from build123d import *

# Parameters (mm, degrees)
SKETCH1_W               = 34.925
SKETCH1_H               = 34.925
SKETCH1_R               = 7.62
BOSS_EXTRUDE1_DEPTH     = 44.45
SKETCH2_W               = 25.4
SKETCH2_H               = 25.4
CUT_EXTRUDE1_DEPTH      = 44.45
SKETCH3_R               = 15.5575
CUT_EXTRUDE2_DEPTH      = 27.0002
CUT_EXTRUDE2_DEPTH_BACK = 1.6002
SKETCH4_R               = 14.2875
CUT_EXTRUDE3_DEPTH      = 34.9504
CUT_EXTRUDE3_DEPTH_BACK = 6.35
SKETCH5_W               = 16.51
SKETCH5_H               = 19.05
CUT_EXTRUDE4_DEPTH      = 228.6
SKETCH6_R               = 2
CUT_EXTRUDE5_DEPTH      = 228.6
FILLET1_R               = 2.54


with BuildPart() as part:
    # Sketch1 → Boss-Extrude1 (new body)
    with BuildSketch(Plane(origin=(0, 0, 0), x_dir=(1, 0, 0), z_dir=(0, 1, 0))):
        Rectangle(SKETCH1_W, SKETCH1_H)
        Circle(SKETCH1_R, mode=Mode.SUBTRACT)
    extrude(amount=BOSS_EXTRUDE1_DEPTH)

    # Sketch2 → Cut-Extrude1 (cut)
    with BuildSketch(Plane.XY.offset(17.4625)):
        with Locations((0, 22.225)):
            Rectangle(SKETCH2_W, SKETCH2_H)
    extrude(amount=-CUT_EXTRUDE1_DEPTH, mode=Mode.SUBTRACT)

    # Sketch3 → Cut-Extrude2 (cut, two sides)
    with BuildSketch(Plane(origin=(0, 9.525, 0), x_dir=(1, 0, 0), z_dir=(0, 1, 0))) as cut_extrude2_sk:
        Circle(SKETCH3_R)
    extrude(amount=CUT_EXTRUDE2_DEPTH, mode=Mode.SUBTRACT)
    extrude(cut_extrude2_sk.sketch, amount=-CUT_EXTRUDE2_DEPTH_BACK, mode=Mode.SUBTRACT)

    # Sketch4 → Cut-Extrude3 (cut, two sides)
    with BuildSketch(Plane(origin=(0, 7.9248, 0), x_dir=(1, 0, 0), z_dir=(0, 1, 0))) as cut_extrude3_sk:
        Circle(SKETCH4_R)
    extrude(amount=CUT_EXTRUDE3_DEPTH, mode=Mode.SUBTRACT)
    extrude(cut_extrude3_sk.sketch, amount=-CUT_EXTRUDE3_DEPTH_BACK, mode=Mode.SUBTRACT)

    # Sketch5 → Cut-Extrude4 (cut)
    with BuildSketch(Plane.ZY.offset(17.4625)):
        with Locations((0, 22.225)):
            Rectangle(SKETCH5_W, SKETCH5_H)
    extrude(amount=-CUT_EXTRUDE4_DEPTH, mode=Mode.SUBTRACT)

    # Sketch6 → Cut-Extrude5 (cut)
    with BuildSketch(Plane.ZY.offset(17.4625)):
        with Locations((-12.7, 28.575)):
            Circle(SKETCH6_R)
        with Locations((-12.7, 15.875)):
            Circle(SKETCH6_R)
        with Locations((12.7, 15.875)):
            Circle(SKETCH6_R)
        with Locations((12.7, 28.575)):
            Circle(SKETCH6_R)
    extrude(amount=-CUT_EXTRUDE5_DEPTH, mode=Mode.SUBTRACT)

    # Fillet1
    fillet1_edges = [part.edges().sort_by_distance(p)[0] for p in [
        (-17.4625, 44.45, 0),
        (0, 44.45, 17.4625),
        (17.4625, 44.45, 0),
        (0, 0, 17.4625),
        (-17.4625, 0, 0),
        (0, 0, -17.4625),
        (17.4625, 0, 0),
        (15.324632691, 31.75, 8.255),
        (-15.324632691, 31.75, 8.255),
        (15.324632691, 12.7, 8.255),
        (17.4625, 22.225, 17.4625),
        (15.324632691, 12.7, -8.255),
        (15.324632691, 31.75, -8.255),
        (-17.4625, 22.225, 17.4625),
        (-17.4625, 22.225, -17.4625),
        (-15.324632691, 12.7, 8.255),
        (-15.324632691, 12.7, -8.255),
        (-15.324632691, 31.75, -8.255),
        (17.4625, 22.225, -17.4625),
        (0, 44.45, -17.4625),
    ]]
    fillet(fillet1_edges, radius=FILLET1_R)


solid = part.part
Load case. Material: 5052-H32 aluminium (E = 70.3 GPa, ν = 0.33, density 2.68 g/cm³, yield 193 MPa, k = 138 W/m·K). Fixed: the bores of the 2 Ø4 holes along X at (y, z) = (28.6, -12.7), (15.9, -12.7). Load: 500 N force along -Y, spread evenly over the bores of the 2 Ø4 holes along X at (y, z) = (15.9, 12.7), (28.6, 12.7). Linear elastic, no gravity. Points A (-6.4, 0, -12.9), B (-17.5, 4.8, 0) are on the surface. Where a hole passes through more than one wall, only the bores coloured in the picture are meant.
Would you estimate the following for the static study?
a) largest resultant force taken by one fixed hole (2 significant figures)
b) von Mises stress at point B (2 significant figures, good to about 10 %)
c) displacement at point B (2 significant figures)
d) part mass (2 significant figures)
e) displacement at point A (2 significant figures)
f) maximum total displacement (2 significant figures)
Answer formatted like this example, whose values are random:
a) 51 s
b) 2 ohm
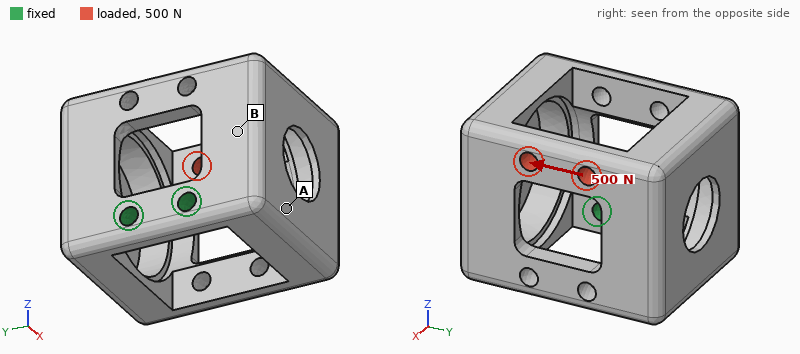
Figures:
a) 670 N
b) 20 MPa
c) 0.044 mm
d) 43 g
e) 0.074 mm
f) 0.19 mm
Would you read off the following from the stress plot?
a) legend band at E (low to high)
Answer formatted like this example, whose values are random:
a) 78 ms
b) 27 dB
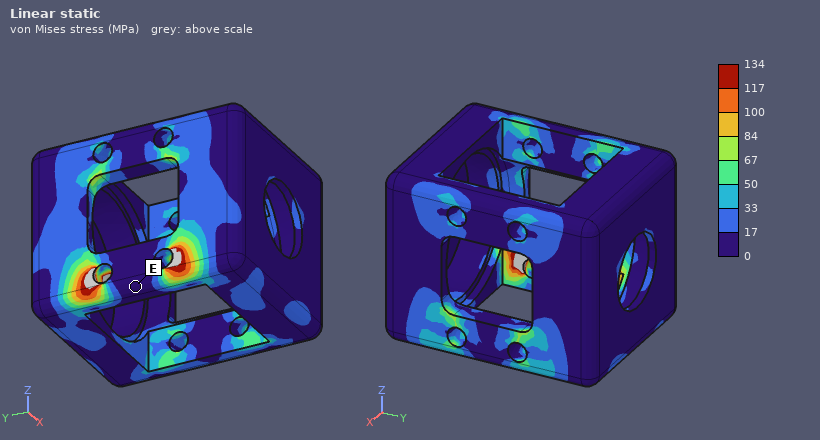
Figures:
a) 0 to 17 MPa
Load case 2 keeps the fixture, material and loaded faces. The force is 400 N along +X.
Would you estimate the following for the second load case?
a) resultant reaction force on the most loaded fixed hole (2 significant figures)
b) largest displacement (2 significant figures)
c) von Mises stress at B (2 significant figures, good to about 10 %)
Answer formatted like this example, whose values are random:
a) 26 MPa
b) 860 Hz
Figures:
a) 210 N
b) 0.26 mm
c) 23 MPa
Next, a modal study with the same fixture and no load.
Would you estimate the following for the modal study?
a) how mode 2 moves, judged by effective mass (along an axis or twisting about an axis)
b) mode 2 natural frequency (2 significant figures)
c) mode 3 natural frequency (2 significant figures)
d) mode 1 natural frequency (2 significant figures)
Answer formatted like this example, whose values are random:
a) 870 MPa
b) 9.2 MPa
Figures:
a) along Y
b) 1900 Hz
c) 3200 Hz
d) 1200 Hz
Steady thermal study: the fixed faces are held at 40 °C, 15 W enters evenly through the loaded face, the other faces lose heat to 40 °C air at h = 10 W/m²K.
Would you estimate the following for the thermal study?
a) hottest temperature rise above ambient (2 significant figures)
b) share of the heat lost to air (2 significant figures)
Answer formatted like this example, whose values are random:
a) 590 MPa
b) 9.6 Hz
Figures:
a) 42 K
b) 13 %
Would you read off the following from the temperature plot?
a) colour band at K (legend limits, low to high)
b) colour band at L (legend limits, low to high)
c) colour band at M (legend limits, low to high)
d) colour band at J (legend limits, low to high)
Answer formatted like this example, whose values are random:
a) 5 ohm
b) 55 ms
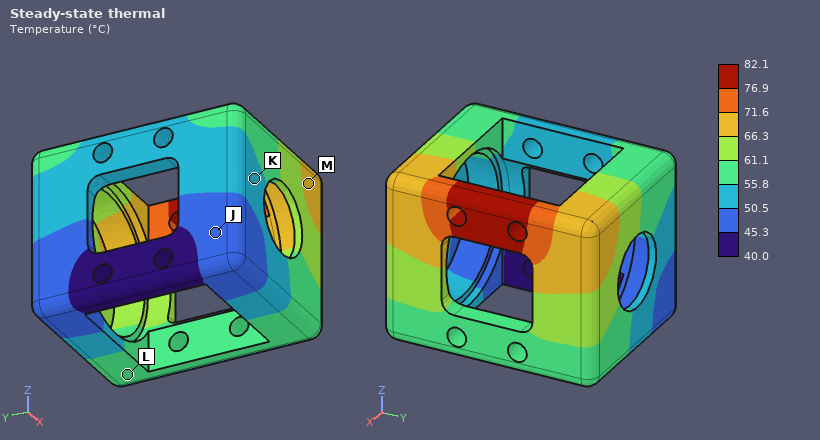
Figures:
a) 50.5 to 55.8 °C
b) 55.8 to 61.1 °C
c) 66.3 to 71.6 °C
d) 45.3 to 50.5 °C
